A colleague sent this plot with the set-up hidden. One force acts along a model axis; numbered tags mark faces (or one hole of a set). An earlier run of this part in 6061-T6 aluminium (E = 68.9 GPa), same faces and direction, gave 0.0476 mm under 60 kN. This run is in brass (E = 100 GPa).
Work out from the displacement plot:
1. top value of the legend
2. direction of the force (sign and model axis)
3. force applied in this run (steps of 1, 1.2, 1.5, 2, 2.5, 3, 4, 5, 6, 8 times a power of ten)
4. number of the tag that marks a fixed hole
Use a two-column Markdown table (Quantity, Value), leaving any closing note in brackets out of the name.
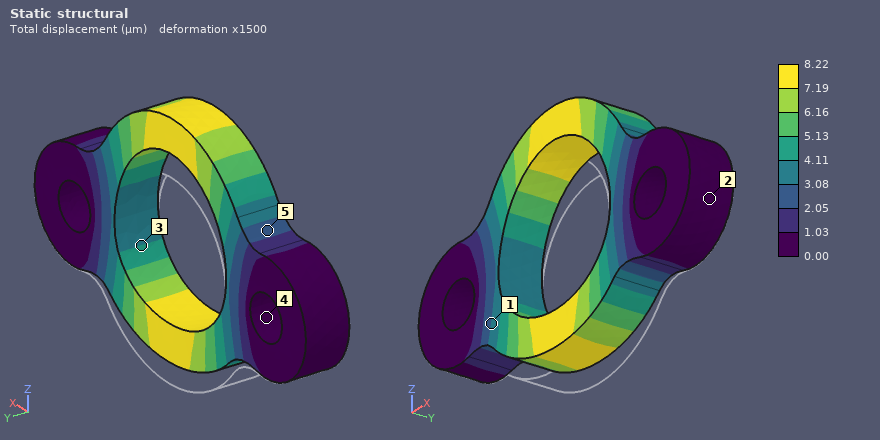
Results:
| Quantity | Value |
|---|---|
| top value of the legend | 8.22 µm |
| direction of the force | +Z |
| force applied in this run | 15 kN |
| number of the tag that marks a fixed hole | 4 |
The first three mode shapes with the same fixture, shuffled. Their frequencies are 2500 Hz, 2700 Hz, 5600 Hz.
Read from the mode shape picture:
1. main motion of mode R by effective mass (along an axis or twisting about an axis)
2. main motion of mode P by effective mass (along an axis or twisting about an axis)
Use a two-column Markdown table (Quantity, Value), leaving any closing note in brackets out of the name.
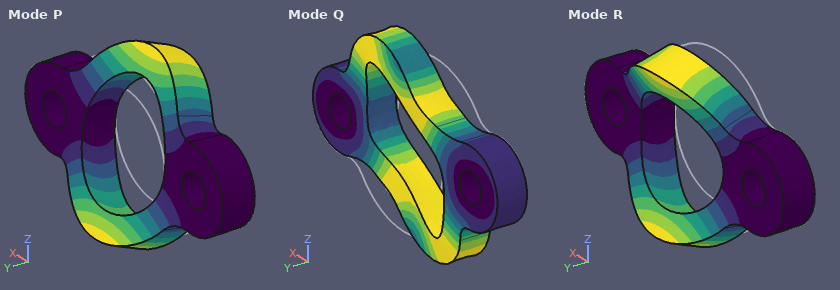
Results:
| Quantity | Value |
|---|---|
| main motion of mode R by effective mass | along Y |
| main motion of mode P by effective mass | twisting about X |
